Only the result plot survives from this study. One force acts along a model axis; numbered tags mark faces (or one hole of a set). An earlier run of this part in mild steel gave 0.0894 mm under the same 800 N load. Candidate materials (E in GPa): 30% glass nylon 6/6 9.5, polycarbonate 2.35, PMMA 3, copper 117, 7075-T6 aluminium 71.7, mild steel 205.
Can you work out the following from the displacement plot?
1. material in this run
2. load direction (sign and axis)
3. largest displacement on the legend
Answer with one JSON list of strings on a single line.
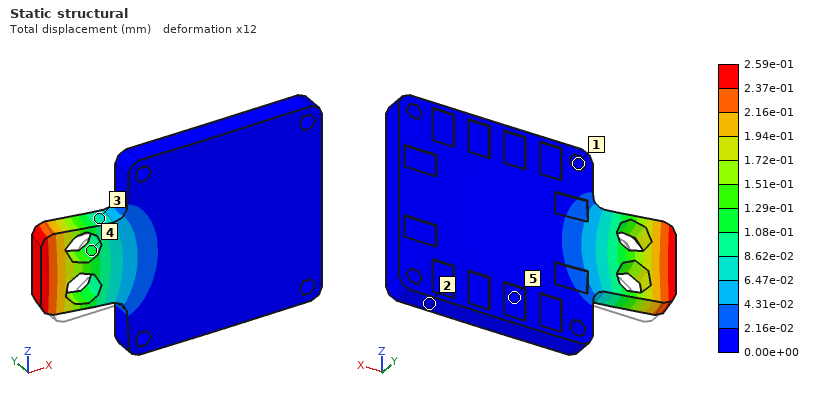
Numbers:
["7075-T6 aluminium", "+Y", "2.59e-01 mm"]
